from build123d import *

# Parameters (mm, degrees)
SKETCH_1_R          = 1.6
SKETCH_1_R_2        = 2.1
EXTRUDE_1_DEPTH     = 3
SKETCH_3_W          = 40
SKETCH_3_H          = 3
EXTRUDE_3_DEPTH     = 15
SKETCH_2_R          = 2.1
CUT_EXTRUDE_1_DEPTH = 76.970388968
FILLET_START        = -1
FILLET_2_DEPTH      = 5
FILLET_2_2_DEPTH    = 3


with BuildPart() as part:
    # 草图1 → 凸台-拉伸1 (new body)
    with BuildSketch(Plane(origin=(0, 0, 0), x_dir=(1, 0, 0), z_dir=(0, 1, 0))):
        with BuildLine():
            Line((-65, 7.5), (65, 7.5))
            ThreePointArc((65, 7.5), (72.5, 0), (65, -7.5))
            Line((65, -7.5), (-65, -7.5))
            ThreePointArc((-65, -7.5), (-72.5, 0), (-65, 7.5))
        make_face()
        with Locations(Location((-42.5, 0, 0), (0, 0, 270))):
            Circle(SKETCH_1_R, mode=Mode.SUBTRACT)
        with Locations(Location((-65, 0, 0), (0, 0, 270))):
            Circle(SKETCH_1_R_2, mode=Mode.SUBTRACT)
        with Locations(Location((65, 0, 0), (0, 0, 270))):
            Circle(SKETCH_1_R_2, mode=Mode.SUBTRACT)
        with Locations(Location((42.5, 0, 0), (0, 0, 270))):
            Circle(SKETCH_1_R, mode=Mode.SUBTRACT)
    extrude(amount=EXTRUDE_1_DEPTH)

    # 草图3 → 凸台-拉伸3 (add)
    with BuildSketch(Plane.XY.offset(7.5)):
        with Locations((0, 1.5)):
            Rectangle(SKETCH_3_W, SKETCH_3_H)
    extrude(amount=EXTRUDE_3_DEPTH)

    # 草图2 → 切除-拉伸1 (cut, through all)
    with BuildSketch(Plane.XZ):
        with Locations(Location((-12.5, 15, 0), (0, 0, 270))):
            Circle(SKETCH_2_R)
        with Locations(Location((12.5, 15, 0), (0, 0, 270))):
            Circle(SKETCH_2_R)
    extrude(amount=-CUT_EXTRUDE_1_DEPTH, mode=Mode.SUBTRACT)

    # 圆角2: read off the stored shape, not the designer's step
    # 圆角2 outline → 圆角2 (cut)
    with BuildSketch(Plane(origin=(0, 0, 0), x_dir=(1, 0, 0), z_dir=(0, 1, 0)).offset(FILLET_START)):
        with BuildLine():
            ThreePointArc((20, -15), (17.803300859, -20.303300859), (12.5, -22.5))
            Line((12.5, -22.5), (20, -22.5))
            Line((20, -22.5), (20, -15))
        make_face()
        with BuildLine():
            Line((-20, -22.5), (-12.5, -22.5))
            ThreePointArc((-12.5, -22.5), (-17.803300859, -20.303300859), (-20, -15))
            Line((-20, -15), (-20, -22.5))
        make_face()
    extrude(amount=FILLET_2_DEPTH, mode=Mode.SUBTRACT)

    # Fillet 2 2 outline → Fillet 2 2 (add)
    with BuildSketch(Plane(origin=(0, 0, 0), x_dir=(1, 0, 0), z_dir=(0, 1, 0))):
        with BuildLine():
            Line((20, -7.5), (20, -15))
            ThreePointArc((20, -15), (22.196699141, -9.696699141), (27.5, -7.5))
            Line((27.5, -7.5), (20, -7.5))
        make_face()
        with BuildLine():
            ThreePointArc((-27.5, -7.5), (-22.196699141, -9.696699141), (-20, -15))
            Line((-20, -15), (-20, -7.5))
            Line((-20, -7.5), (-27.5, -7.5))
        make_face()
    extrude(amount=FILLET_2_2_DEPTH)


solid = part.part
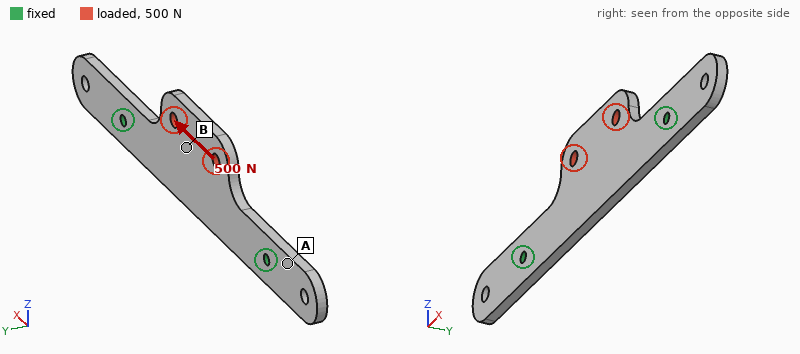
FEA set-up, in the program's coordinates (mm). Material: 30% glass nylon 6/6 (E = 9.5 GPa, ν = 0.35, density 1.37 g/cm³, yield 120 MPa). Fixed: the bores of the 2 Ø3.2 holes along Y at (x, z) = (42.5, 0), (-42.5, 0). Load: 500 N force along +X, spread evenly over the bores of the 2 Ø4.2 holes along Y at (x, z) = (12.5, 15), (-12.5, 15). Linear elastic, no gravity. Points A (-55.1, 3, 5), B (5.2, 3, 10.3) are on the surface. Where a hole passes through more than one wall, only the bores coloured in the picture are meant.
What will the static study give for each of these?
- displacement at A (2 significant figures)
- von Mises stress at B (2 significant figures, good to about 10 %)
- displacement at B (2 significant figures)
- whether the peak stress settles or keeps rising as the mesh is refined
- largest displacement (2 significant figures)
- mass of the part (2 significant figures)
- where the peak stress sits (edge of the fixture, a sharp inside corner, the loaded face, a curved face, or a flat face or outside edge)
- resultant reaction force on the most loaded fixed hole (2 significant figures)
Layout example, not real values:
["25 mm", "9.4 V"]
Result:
["11 µm", "4.8 MPa", "33 µm", "keeps rising", "54 µm", "11 g", "edge of the fixture", "270 N"]
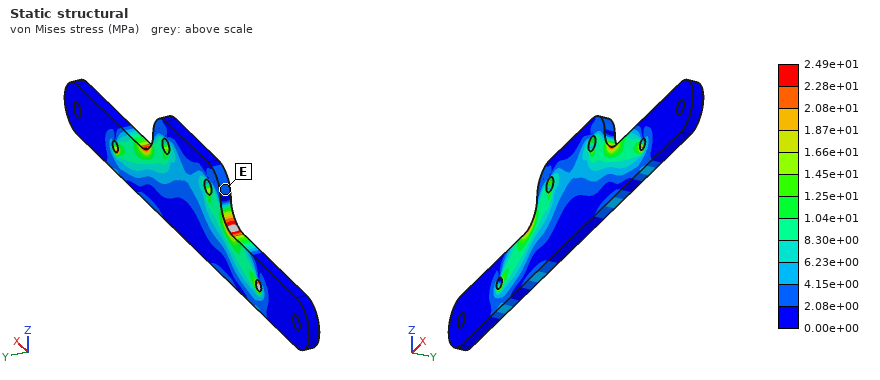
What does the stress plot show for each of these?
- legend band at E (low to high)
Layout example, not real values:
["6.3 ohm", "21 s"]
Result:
["2.08e+00 to 4.15e+00 MPa"]
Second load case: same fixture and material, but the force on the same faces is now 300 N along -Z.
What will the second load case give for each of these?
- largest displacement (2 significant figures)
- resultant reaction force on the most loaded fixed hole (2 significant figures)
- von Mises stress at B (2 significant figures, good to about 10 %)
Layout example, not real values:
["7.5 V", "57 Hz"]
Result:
["0.11 mm", "180 N", "5.0 MPa"]
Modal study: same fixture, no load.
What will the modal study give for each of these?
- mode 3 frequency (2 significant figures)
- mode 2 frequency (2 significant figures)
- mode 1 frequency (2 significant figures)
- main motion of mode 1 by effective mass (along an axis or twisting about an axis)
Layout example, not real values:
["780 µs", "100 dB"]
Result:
["1600 Hz", "1600 Hz", "830 Hz", "along Y"]
